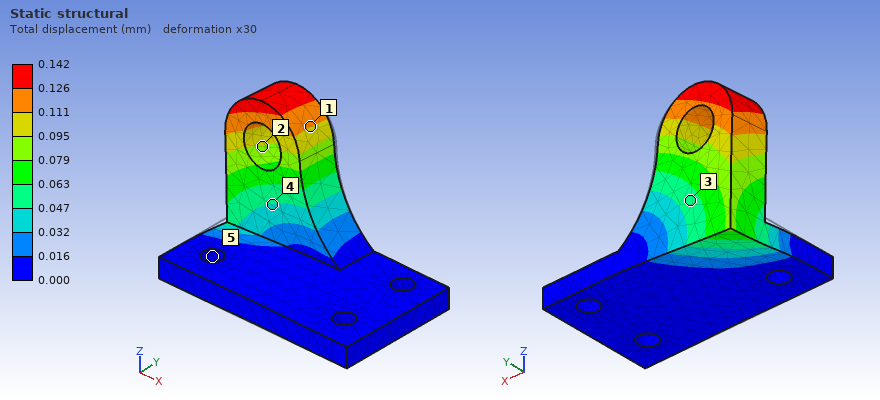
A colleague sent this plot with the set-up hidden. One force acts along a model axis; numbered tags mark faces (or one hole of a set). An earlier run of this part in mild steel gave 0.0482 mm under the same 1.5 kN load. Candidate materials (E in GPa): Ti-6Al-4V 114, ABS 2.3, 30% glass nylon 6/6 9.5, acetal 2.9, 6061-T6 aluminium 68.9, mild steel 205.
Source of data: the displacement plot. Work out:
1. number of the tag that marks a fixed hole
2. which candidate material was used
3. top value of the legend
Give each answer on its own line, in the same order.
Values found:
5
6061-T6 aluminium
0.142 mm
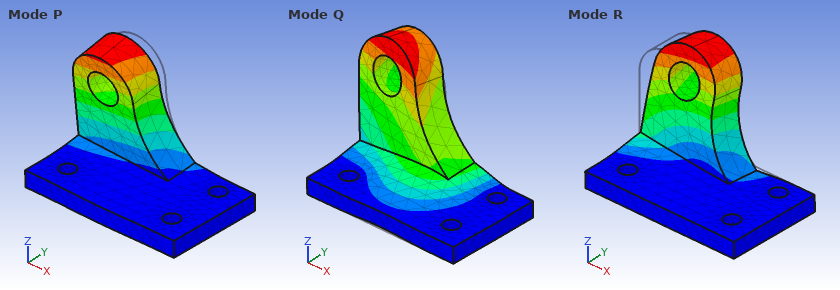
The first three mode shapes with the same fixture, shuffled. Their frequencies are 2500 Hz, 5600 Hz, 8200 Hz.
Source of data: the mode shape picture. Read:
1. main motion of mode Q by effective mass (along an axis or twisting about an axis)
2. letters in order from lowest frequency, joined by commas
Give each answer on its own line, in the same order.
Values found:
along Z
P, R, Q
